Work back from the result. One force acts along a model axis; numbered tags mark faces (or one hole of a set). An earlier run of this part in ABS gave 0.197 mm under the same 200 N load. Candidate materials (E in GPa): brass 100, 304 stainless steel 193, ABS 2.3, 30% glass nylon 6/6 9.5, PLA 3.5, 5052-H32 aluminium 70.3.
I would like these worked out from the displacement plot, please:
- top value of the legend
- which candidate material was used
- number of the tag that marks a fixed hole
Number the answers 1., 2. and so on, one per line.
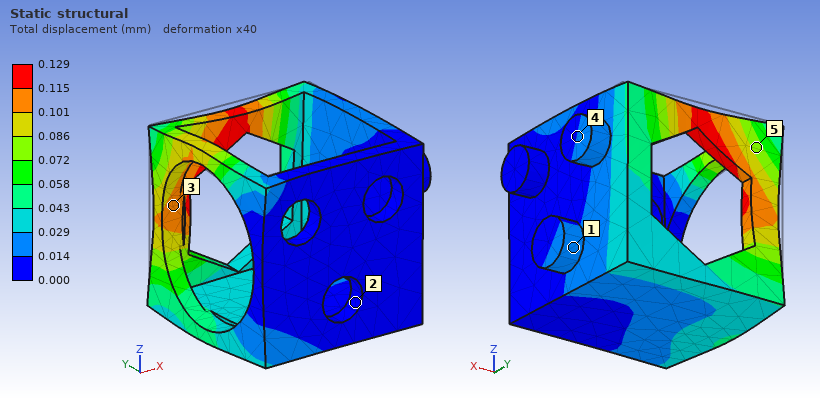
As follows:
1. 0.129 mm
2. PLA
3. 2
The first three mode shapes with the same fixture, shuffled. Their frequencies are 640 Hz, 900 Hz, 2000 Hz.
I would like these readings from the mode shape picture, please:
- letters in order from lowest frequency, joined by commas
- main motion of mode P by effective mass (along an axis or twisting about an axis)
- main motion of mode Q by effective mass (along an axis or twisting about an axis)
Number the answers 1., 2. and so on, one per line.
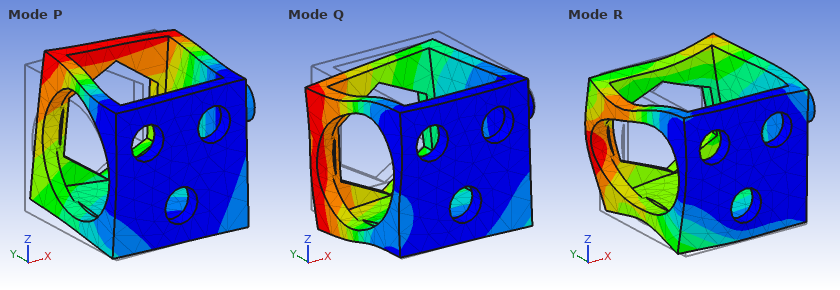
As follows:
1. P, Q, R
2. along X
3. along Z
